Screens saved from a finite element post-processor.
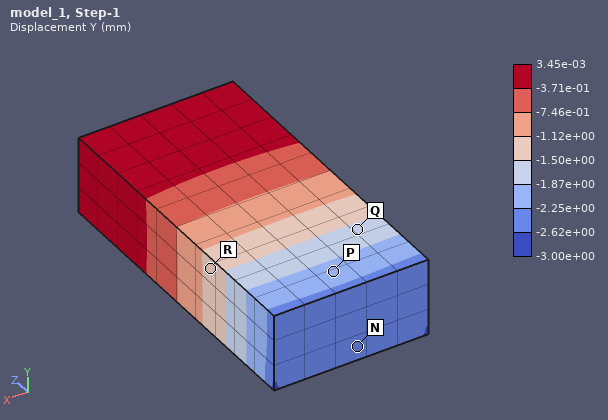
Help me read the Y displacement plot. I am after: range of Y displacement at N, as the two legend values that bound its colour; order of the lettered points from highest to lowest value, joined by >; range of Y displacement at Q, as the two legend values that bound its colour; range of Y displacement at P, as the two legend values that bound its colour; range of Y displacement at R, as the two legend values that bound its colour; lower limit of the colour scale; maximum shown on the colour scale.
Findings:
-2.62e+00 to -2.25e+00 mm
R > Q > P > N
-1.87e+00 to -1.50e+00 mm
-2.25e+00 to -1.87e+00 mm
-1.50e+00 to -1.12e+00 mm
-3.00e+00 mm
3.45e-03 mm
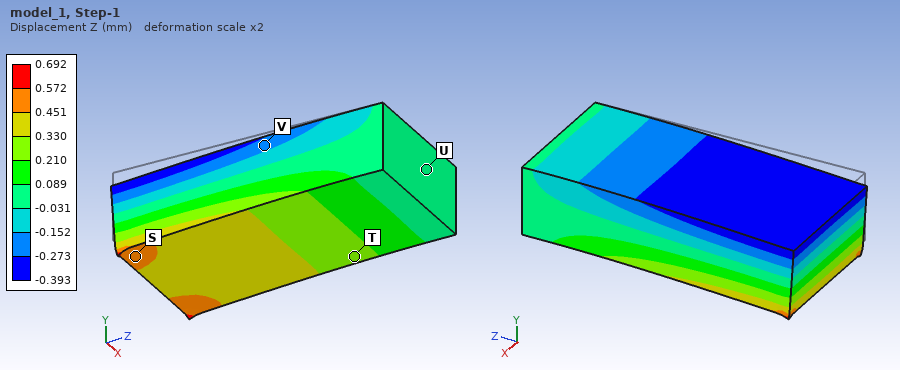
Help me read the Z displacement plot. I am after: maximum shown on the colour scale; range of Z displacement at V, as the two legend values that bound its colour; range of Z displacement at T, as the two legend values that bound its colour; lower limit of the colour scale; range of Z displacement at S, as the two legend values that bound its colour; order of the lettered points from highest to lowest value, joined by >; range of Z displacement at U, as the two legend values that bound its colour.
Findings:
0.692 mm
-0.273 to -0.152 mm
0.210 to 0.330 mm
-0.393 mm
0.451 to 0.572 mm
S > T > U > V
-0.031 to 0.089 mm
